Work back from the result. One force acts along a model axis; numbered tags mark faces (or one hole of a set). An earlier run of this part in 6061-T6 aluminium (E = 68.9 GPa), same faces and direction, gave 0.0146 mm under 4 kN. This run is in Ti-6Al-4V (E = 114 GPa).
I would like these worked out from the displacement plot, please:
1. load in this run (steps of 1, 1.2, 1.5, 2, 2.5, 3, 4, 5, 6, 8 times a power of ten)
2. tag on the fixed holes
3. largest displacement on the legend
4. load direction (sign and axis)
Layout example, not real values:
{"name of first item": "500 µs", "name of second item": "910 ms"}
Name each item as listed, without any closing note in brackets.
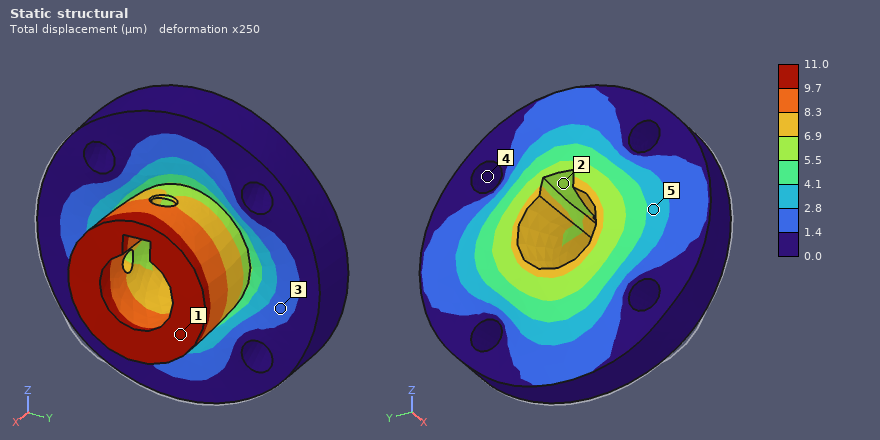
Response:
{"load in this run": "5 kN", "tag on the fixed holes": "4", "largest displacement on the legend": "11.0 µm", "load direction": "-X"}
